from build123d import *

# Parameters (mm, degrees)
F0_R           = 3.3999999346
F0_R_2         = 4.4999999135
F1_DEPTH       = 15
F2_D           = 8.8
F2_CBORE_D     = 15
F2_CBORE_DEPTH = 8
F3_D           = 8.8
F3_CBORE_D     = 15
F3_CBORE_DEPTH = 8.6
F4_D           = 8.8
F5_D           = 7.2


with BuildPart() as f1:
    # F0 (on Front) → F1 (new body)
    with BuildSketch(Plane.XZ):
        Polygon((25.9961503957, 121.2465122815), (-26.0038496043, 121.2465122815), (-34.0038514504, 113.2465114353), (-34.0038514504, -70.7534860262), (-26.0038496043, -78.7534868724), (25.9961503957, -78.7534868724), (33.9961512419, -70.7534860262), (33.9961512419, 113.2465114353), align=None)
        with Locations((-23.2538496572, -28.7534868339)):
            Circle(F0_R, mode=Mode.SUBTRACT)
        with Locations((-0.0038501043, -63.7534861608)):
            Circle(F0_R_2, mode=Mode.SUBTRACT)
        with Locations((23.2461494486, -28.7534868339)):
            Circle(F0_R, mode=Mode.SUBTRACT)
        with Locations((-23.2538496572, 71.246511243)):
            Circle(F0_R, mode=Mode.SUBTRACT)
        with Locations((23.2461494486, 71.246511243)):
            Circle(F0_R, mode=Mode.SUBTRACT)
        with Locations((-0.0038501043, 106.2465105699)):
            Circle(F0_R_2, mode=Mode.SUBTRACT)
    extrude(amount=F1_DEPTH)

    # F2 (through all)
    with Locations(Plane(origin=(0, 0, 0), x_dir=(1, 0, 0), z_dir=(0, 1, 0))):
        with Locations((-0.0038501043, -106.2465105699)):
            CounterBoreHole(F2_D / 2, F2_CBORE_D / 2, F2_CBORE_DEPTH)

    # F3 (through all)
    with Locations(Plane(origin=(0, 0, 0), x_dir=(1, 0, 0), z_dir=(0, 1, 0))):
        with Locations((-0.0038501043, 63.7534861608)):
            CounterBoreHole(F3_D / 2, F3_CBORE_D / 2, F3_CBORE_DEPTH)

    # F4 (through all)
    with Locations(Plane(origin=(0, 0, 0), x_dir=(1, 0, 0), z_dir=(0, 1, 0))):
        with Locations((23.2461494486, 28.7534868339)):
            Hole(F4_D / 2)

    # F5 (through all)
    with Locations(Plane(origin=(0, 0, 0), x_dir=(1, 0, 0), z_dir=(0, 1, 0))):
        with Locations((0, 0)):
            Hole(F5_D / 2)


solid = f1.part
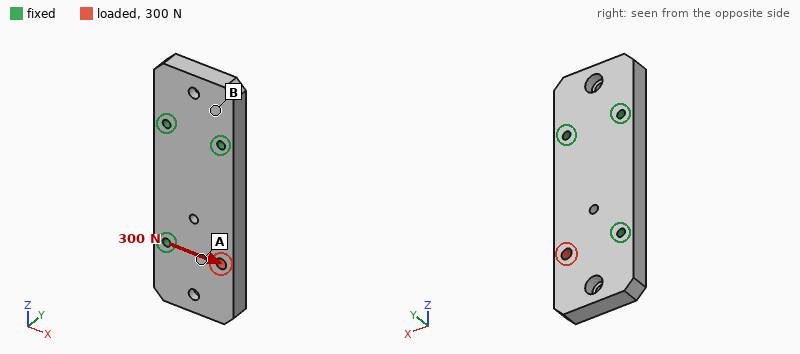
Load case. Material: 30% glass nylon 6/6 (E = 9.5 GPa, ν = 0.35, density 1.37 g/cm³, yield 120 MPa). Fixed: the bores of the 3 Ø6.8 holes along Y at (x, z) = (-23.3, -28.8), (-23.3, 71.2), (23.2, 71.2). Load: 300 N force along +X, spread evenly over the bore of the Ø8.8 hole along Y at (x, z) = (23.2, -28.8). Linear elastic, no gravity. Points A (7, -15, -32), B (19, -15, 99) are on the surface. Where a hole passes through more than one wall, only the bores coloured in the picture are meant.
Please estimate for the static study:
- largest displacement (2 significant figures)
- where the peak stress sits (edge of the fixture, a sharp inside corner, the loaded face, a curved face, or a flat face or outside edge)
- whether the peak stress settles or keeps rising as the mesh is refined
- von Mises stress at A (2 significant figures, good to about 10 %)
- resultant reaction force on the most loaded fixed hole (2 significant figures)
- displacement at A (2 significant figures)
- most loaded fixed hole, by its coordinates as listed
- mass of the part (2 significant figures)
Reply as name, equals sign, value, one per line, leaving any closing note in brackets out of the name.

largest displacement = 4.6 µm
where the peak stress sits = edge of the fixture
whether the peak stress settles or keeps rising as the mesh is refined = keeps rising
von Mises stress at A = 0.68 MPa
resultant reaction force on the most loaded fixed hole = 280 N
displacement at A = 2.3 µm
most loaded fixed hole, by its coordinates as listed = (-23.3, -28.8)
mass of the part = 270 g
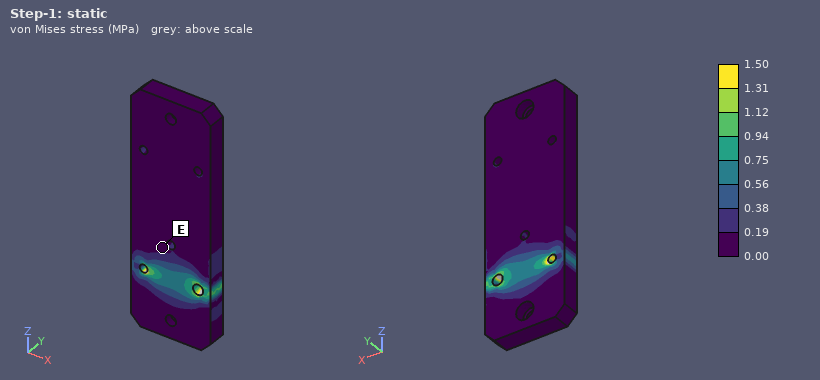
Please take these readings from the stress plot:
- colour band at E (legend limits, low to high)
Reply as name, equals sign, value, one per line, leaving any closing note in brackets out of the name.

colour band at E = 0.00 to 0.19 MPa
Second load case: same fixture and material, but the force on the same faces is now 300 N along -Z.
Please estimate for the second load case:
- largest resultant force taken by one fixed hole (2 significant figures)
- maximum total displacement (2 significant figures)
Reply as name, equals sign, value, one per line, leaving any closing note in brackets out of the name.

largest resultant force taken by one fixed hole = 130 N
maximum total displacement = 8.1 µm
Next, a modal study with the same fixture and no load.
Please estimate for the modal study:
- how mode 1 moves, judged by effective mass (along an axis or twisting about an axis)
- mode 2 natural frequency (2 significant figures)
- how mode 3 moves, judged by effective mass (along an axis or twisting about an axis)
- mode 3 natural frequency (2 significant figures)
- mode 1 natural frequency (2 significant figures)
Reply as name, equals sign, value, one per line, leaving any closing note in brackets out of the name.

how mode 1 moves, judged by effective mass = along Y
mode 2 natural frequency = 2100 Hz
how mode 3 moves, judged by effective mass = along Y
mode 3 natural frequency = 2400 Hz
mode 1 natural frequency = 1400 Hz
